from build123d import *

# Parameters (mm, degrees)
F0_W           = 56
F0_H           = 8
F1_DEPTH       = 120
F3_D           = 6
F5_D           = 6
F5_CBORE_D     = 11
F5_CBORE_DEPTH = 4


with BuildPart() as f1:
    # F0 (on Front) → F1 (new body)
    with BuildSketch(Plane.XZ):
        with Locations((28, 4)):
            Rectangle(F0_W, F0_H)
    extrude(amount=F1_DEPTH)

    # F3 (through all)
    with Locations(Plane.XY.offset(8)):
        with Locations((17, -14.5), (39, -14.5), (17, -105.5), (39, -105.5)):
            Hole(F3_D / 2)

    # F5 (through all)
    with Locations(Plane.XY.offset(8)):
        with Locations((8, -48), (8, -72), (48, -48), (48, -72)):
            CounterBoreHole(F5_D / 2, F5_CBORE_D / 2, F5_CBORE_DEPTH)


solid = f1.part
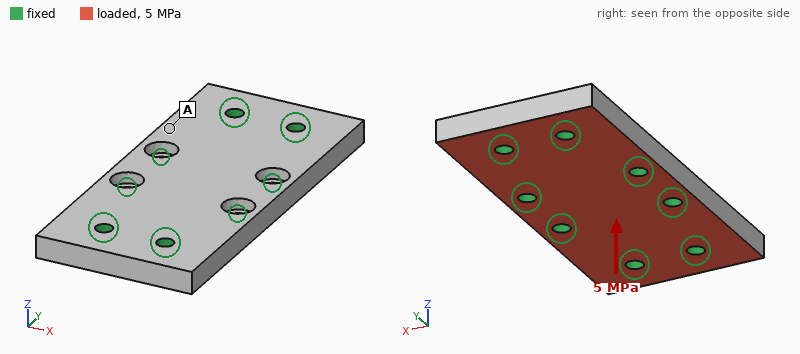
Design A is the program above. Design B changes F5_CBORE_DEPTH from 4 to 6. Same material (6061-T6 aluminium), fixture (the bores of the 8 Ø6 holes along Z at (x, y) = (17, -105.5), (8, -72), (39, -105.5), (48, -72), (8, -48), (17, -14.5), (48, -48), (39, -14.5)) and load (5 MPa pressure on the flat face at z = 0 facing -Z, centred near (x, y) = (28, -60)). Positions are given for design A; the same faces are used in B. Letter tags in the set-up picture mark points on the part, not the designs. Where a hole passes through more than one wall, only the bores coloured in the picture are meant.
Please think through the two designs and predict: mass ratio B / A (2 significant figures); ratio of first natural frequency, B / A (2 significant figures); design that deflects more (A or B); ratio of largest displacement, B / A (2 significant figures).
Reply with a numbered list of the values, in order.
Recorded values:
1. 0.99
2. 0.85
3. B
4. 1.4
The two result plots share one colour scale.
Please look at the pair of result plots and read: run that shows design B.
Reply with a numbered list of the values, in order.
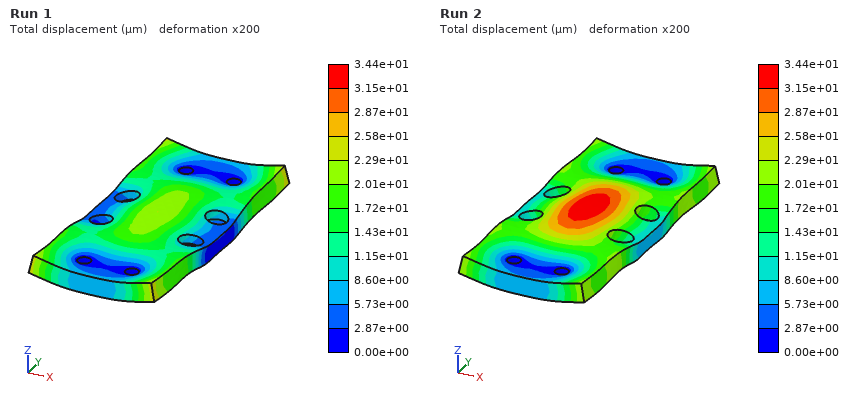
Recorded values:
1. Run 2
